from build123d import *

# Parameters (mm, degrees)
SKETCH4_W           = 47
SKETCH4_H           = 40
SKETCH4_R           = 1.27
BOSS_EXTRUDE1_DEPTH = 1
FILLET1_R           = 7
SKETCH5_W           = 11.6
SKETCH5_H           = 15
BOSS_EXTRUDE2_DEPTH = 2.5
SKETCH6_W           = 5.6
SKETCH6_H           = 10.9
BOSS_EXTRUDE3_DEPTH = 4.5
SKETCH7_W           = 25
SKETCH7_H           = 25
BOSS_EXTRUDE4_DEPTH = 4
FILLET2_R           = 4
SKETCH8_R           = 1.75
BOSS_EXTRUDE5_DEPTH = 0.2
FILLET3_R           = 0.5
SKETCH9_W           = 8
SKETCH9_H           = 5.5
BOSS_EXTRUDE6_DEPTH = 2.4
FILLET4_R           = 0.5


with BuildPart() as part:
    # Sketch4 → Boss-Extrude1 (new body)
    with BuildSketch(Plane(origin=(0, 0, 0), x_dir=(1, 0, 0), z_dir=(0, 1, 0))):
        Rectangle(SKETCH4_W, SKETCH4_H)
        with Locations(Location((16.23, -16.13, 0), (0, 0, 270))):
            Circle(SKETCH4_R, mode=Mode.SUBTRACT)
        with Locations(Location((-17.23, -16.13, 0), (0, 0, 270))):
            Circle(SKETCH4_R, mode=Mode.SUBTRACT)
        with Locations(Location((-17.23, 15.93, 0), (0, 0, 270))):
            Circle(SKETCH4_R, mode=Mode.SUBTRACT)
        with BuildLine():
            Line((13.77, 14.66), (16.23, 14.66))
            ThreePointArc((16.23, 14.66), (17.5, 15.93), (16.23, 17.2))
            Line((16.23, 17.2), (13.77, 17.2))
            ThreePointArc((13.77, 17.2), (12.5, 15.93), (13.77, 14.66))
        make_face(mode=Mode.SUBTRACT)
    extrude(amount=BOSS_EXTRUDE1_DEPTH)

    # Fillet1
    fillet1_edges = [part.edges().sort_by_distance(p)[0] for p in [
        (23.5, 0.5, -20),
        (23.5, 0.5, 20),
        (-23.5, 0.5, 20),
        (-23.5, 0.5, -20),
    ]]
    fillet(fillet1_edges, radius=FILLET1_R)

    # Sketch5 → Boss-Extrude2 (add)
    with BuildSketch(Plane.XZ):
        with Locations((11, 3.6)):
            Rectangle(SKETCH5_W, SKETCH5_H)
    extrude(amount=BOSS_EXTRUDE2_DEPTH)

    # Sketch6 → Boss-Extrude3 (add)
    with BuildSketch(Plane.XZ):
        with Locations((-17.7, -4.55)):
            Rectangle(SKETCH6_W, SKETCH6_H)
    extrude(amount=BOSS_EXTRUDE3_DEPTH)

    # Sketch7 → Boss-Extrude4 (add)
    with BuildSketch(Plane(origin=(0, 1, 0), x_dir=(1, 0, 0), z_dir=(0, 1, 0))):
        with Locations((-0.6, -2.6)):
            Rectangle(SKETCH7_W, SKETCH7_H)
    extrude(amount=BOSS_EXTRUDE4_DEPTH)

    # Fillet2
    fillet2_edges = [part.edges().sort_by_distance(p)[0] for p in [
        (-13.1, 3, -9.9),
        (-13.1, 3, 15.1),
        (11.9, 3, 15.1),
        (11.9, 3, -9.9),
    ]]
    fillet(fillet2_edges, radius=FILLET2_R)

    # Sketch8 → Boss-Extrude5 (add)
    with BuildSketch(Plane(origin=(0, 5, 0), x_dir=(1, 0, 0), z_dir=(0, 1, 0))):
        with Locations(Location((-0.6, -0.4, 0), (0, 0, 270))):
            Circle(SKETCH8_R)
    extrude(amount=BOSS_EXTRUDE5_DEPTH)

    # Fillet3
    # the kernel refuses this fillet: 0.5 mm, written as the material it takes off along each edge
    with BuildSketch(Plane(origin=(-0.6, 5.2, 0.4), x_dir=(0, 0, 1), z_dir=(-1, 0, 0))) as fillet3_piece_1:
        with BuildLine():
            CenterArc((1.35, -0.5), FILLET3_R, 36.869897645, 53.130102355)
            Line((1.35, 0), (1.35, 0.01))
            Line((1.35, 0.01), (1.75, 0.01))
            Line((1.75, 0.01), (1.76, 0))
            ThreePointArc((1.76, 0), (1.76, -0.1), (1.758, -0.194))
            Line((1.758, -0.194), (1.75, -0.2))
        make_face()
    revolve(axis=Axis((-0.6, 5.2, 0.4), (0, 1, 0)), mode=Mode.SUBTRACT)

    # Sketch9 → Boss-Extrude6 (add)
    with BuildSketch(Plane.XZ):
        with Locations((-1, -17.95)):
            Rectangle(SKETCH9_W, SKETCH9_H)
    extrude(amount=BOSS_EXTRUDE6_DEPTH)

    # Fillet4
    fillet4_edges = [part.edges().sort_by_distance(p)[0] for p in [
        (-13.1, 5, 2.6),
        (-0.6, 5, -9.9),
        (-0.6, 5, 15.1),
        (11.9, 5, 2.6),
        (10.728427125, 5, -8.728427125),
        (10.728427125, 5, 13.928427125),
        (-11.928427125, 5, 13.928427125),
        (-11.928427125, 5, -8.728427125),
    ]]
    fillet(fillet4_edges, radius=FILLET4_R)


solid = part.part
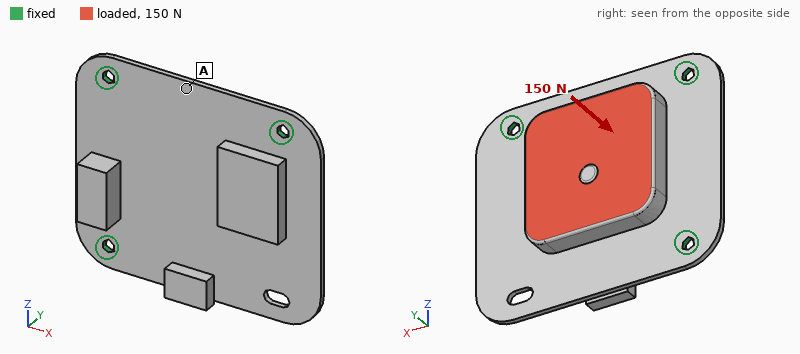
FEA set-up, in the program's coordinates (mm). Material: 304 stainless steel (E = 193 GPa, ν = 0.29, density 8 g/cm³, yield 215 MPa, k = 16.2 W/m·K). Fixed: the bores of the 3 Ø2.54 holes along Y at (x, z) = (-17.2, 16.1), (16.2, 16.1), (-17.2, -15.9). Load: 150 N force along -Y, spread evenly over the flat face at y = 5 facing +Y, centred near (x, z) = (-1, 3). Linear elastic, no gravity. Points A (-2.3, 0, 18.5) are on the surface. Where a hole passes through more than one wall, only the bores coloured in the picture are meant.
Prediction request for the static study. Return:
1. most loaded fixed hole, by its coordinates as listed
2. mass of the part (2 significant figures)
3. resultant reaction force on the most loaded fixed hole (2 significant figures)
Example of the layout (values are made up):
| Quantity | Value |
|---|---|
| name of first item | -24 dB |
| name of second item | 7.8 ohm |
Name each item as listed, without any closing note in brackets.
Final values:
| Quantity | Value |
|---|---|
| most loaded fixed hole, by its coordinates as listed | (16.2, 16.1) |
| mass of the part | 41 g |
| resultant reaction force on the most loaded fixed hole | 86 N |
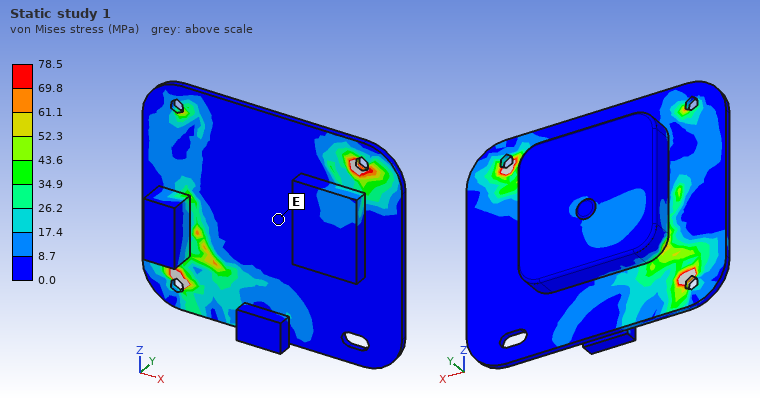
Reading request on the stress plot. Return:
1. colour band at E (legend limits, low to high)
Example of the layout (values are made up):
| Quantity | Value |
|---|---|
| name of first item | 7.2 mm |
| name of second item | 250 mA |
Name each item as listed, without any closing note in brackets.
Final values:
| Quantity | Value |
|---|---|
| colour band at E | 0.0 to 8.7 MPa |
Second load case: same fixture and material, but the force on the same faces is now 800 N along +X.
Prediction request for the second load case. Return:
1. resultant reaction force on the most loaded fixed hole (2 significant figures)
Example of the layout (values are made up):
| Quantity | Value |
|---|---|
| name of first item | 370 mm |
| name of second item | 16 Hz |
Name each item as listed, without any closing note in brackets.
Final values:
| Quantity | Value |
|---|---|
| resultant reaction force on the most loaded fixed hole | 350 N |
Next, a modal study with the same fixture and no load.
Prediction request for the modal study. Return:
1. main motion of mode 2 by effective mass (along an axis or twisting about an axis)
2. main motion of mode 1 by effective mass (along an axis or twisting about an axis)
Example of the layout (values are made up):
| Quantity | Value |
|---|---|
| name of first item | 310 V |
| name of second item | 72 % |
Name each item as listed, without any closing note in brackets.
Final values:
| Quantity | Value |
|---|---|
| main motion of mode 2 by effective mass | along Y |
| main motion of mode 1 by effective mass | along Y |
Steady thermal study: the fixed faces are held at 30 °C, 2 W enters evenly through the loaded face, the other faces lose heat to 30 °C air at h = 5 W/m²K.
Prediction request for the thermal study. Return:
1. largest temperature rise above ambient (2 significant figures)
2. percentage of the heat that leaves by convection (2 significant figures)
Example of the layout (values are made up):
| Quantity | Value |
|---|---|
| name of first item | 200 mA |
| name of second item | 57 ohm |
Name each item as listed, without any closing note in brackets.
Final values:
| Quantity | Value |
|---|---|
| largest temperature rise above ambient | 23 K |
| percentage of the heat that leaves by convection | 17 % |
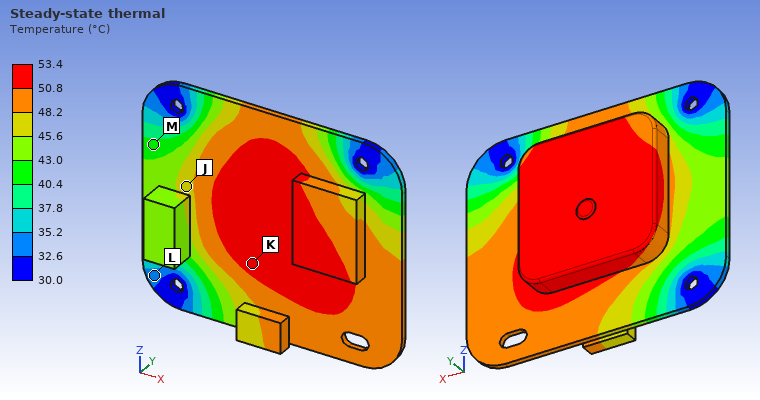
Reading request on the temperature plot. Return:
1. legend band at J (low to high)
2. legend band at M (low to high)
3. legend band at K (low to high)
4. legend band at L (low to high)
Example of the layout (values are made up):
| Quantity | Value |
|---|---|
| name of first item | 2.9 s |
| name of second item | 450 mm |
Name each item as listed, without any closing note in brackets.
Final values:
| Quantity | Value |
|---|---|
| legend band at J | 45.6 to 48.2 °C |
| legend band at M | 40.4 to 43.0 °C |
| legend band at K | 50.8 to 53.4 °C |
| legend band at L | 32.6 to 35.2 °C |
